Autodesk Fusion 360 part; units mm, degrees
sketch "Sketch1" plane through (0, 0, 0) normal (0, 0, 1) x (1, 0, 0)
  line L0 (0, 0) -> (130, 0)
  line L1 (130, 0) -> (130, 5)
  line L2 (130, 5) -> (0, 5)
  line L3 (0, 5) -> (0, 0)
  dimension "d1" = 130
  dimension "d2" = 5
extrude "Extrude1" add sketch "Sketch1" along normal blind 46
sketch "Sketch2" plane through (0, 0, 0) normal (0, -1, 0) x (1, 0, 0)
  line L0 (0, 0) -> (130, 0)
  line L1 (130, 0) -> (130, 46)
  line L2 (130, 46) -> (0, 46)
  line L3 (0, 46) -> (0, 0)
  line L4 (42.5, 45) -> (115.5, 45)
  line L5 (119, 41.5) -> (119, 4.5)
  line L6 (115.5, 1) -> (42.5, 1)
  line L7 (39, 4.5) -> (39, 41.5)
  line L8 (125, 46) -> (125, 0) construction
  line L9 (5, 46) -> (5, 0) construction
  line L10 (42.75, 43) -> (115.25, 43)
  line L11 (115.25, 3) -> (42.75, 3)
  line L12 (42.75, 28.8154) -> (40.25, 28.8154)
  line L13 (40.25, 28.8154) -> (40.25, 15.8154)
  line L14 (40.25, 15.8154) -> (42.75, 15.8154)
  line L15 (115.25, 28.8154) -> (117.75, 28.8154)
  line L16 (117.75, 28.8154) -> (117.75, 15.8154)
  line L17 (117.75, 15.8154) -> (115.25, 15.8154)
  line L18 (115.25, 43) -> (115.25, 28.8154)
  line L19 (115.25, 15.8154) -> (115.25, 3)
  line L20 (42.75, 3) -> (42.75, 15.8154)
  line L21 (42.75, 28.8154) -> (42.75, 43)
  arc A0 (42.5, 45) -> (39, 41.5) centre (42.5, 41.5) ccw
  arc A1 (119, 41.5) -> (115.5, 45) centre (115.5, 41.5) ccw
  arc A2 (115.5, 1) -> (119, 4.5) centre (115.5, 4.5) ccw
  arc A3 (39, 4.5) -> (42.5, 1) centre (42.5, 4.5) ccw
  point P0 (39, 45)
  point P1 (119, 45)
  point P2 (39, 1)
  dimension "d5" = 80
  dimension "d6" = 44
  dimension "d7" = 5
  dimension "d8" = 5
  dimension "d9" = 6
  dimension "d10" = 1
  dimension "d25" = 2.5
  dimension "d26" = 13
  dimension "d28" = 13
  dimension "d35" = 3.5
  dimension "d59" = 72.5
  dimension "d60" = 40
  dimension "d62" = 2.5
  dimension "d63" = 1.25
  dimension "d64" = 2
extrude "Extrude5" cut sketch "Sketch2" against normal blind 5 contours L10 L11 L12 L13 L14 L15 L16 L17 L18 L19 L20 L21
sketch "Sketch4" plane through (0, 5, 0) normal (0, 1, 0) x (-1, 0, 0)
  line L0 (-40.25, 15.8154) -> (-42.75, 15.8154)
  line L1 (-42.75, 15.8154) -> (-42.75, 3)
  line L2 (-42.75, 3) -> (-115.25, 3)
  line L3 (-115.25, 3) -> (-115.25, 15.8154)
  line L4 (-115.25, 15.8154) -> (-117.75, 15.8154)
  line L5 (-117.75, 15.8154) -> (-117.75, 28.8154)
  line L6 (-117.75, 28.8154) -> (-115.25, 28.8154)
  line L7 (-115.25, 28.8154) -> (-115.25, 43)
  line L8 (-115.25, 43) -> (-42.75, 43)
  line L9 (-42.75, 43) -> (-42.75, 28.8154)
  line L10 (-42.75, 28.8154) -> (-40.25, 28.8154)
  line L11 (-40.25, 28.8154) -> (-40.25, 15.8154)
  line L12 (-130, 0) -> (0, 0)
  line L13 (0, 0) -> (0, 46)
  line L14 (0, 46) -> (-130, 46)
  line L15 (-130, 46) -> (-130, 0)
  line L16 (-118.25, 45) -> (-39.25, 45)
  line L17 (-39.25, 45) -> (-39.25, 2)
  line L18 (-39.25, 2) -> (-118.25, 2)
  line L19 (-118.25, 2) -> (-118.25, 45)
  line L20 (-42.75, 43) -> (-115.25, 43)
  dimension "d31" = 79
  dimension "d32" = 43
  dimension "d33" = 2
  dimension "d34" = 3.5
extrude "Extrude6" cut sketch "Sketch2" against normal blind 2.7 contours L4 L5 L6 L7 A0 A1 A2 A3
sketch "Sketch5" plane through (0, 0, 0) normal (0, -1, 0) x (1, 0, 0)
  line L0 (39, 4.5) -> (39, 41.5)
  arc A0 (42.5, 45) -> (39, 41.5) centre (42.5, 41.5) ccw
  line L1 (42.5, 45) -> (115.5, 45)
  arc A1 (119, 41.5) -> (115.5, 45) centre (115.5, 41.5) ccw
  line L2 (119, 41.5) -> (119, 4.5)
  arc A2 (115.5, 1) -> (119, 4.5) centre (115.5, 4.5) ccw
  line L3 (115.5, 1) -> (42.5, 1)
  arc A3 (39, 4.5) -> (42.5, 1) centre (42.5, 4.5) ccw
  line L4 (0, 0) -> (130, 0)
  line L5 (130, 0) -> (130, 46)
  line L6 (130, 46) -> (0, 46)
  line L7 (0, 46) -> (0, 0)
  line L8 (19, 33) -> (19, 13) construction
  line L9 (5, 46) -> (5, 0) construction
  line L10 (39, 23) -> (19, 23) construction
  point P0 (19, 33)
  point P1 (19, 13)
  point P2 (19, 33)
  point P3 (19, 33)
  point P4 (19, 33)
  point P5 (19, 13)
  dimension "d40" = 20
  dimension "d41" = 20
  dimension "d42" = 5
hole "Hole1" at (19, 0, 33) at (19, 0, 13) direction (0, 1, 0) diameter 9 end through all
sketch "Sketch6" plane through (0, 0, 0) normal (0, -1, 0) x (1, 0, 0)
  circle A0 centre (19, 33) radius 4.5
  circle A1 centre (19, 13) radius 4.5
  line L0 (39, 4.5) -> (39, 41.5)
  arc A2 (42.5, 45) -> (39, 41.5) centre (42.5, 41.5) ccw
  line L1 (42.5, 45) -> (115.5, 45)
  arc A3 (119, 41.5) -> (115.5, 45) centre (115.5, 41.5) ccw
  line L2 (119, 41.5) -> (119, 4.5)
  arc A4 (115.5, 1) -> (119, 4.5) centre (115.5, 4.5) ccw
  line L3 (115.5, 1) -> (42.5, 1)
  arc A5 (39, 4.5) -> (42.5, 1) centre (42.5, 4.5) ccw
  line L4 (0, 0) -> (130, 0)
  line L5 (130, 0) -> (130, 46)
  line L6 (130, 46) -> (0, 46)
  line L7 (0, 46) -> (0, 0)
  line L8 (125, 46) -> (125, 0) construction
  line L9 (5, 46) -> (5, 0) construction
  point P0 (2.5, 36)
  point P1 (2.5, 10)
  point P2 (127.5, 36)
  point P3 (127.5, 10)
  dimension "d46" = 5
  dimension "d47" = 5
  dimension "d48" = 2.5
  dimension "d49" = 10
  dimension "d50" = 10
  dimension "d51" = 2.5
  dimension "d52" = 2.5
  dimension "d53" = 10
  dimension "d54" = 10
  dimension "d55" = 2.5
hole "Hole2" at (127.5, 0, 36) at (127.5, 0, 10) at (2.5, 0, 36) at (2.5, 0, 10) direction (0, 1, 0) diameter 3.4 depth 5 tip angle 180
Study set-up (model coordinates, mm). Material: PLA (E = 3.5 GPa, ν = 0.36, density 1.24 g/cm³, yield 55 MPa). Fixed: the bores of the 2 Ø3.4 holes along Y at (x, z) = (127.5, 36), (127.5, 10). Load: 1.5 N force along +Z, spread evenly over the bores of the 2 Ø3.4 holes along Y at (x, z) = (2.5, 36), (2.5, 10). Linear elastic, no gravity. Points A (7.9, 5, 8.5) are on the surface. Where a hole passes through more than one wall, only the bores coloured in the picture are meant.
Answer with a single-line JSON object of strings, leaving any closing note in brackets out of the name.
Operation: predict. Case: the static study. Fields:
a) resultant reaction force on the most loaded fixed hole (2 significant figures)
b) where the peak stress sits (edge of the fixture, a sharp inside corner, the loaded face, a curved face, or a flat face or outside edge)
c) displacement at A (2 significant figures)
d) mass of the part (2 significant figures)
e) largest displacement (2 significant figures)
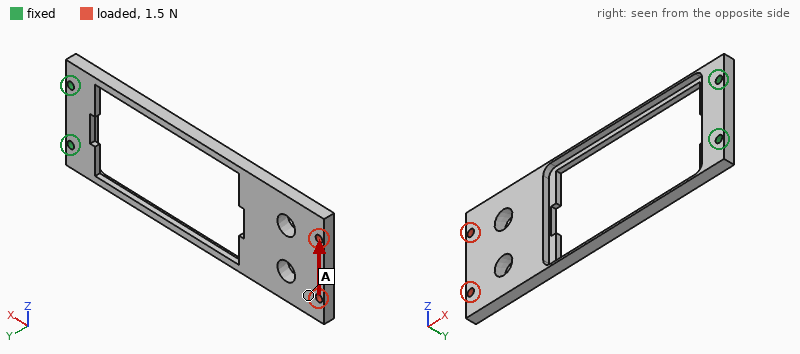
{"resultant reaction force on the most loaded fixed hole": "5.7 N", "where the peak stress sits": "a flat face or outside edge", "displacement at A": "1.3 mm", "mass of the part": "16 g", "largest displacement": "1.4 mm"}
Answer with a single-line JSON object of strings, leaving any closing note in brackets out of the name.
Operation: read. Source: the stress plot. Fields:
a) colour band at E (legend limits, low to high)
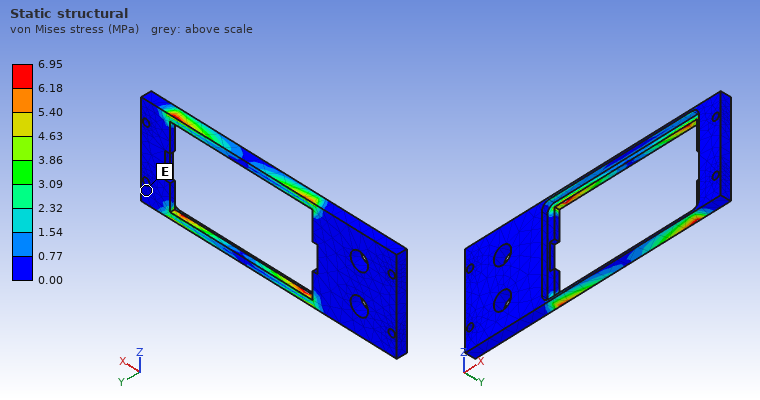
{"colour band at E": "0.00 to 0.77 MPa"}
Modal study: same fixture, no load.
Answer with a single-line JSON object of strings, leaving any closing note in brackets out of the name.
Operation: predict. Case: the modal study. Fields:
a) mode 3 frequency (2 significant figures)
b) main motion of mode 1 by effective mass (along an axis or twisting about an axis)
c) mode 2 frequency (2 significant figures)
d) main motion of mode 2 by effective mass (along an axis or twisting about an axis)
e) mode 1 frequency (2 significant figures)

{"mode 3 frequency": "130 Hz", "main motion of mode 1 by effective mass": "along Y", "mode 2 frequency": "49 Hz", "main motion of mode 2 by effective mass": "along Z", "mode 1 frequency": "28 Hz"}
